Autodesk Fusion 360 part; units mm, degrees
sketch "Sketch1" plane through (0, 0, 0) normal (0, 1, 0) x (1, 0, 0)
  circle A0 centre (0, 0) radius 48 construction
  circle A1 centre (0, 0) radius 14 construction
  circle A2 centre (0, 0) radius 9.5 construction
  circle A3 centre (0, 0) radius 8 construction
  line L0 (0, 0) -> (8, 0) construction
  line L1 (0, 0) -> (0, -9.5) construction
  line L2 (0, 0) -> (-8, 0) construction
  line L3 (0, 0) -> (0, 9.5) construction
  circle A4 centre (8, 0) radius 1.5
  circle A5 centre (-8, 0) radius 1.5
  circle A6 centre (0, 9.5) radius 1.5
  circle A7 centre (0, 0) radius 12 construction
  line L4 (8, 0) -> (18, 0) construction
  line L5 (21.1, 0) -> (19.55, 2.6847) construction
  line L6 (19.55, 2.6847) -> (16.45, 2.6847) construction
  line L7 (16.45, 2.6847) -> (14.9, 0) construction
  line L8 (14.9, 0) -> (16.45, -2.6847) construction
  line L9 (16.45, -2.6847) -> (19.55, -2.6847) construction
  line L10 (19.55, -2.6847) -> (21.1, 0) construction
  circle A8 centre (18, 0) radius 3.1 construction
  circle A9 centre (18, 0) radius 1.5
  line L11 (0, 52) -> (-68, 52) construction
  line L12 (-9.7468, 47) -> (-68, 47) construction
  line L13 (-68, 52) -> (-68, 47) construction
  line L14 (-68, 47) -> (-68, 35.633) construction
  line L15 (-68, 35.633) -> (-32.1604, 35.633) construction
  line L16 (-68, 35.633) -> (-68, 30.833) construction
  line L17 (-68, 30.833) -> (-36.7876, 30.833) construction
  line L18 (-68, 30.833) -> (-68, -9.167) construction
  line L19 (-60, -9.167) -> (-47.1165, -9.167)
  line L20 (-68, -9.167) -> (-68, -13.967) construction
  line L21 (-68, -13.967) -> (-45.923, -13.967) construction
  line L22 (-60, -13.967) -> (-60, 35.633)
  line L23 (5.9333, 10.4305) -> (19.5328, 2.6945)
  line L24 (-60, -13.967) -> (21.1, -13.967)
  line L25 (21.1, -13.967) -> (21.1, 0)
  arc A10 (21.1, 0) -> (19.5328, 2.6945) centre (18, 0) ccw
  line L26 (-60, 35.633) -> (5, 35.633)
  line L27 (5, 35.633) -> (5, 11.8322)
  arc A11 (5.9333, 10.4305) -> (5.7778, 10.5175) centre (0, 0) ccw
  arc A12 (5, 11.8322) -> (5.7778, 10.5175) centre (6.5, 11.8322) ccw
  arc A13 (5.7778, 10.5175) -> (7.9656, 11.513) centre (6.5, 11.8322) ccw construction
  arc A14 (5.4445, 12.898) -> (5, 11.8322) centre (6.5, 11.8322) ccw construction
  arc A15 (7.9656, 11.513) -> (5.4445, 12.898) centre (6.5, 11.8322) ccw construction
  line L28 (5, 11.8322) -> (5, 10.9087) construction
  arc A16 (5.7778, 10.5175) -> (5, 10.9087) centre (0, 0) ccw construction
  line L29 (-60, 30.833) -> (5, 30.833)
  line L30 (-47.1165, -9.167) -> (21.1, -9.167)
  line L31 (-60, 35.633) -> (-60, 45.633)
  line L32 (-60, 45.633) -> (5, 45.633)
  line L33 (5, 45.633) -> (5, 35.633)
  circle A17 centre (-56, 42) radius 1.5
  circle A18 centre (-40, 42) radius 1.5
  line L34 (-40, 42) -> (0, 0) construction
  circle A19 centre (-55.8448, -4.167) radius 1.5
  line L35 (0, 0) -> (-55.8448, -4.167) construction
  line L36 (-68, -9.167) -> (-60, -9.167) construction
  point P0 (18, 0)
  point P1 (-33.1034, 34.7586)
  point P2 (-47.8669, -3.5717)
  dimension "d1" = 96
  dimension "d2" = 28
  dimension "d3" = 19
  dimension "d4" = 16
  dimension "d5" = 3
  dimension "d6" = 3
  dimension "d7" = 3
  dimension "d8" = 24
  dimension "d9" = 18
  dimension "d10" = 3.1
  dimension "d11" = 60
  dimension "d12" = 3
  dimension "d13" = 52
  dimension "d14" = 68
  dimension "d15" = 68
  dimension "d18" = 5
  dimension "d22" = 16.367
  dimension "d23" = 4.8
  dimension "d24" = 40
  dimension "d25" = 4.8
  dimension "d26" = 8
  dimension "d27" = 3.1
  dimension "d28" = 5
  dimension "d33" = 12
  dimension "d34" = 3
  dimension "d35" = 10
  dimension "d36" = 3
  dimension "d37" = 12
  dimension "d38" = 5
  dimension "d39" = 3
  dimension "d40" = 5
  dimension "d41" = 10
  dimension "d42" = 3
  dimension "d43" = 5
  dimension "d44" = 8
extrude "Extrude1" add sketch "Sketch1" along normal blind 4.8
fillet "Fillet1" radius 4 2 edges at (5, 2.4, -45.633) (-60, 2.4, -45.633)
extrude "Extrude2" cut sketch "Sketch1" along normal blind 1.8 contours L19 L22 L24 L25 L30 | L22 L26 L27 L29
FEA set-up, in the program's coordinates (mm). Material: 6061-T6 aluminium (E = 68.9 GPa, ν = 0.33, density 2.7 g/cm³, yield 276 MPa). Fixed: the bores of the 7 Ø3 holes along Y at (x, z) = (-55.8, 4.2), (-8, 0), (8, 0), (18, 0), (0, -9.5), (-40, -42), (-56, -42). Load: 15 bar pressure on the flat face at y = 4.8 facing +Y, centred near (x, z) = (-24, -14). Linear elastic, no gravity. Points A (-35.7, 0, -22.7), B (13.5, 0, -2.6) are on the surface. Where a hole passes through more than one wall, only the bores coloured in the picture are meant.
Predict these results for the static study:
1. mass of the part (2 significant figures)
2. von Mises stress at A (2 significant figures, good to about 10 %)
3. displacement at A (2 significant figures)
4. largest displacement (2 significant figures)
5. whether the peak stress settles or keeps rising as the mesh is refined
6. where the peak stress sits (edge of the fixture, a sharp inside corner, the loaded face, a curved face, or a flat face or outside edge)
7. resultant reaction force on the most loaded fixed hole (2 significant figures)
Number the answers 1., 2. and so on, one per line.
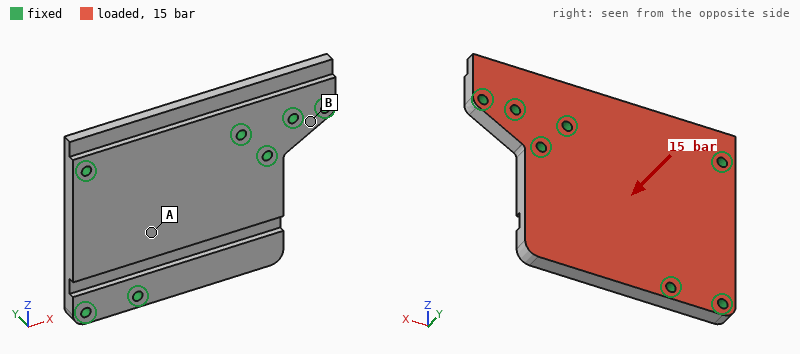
1. 50 g
2. 41 MPa
3. 0.060 mm
4. 0.27 mm
5. keeps rising
6. edge of the fixture
7. 1.6 kN
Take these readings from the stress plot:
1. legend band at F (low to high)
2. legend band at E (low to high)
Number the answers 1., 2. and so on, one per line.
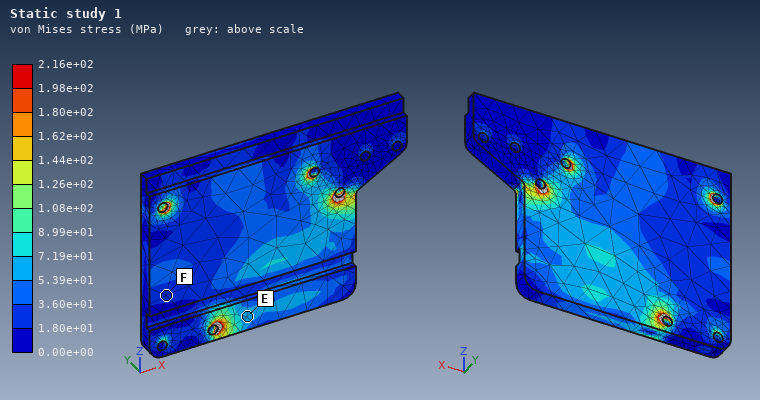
1. 1.80e+01 to 3.60e+01 MPa
2. 5.39e+01 to 7.19e+01 MPa
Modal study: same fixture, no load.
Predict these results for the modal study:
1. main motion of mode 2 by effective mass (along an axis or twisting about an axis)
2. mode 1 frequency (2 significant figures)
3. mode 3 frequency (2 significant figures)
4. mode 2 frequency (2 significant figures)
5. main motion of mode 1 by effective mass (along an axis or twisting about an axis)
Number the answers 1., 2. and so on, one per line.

1. along Y
2. 4600 Hz
3. 10 kHz
4. 8200 Hz
5. along Y
